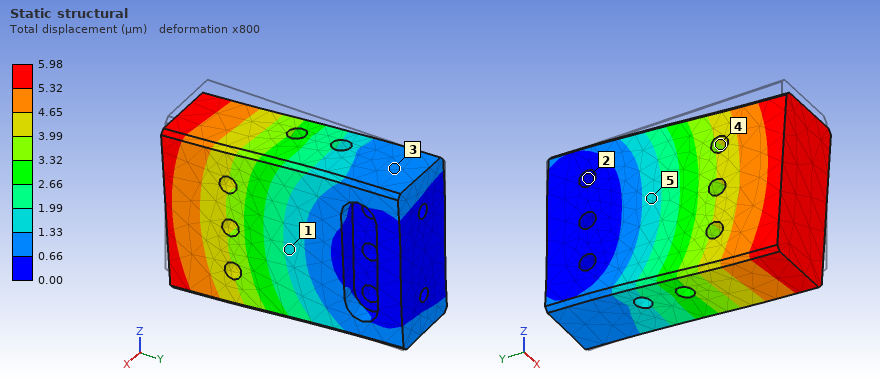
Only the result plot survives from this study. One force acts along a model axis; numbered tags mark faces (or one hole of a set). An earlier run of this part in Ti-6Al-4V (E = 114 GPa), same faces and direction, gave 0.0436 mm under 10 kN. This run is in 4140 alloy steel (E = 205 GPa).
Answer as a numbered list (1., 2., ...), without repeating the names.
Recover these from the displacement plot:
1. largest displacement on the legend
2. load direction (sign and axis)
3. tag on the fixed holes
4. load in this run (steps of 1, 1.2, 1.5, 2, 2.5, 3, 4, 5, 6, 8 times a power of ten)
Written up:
1. 5.98 µm
2. -Z
3. 2
4. 2.5 kN
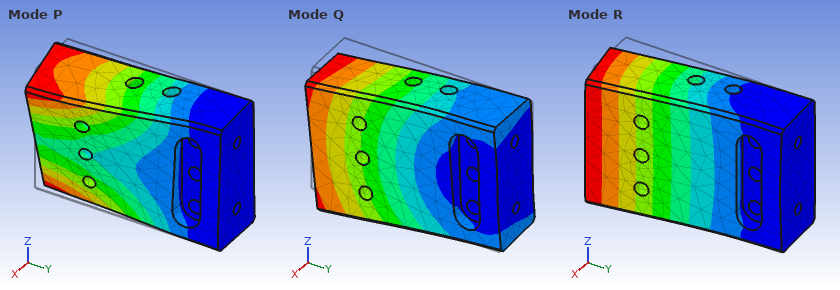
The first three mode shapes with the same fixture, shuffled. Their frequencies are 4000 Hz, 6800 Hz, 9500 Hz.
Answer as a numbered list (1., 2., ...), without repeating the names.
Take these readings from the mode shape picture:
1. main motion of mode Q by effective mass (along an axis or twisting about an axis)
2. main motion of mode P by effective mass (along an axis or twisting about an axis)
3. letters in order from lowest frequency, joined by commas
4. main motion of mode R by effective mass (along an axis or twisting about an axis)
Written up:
1. along Z
2. twisting about Y
3. R, Q, P
4. along X
